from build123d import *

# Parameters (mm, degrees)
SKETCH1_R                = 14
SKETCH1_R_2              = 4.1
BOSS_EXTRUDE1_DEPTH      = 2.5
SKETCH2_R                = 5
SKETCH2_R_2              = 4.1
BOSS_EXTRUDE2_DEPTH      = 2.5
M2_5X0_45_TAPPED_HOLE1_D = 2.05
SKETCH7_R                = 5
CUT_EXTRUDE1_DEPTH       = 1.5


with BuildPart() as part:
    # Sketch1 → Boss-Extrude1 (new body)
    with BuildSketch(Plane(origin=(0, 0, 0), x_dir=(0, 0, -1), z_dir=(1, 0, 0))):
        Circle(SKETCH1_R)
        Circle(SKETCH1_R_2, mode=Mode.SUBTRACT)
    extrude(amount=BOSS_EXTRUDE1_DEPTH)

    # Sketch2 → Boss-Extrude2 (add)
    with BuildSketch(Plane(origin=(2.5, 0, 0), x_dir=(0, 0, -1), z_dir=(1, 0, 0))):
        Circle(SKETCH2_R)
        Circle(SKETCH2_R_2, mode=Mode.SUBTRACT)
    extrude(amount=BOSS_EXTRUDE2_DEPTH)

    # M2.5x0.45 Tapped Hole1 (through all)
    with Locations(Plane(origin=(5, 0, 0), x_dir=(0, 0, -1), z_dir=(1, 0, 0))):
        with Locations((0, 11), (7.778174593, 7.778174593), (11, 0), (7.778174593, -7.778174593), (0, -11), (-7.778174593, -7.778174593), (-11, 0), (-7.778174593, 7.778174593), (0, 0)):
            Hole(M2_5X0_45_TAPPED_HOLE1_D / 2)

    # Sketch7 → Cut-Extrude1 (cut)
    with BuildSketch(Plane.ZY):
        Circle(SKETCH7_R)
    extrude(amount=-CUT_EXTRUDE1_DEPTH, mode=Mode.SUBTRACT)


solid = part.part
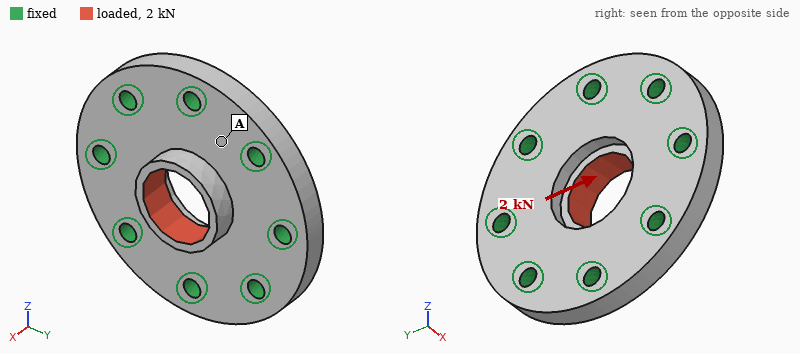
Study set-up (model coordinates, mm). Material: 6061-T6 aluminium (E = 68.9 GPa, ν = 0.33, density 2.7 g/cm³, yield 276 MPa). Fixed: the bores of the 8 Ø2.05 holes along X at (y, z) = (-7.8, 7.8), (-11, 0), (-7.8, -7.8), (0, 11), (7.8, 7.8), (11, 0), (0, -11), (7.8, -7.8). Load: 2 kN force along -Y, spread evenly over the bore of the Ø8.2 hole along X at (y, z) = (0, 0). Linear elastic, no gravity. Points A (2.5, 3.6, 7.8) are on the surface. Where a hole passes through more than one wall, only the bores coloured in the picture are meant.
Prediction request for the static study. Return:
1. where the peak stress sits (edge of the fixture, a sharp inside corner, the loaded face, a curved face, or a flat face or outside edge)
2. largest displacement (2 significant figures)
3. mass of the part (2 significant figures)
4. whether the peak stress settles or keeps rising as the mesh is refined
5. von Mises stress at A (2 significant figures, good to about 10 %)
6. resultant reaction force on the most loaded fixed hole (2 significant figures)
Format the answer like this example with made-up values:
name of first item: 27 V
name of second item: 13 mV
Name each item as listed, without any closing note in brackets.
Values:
where the peak stress sits: a sharp inside corner
largest displacement: 19 µm
mass of the part: 3.7 g
whether the peak stress settles or keeps rising as the mesh is refined: keeps rising
von Mises stress at A: 22 MPa
resultant reaction force on the most loaded fixed hole: 410 N
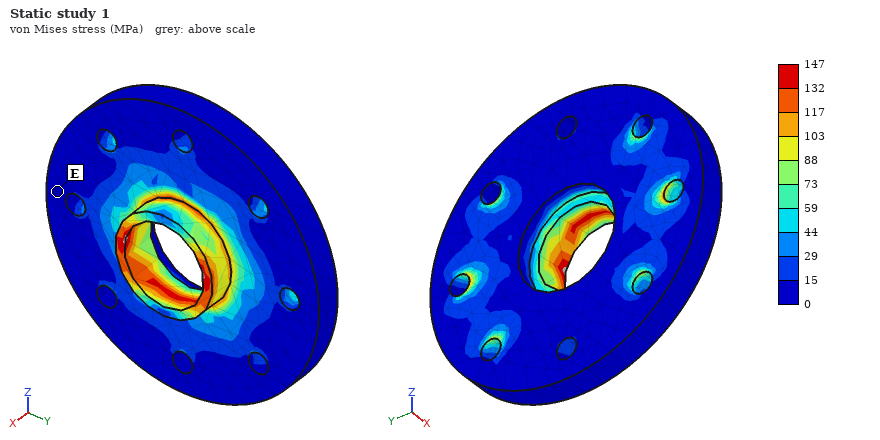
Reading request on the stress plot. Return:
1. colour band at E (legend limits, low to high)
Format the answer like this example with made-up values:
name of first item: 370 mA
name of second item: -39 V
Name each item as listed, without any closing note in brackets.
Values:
colour band at E: 0 to 15 MPa
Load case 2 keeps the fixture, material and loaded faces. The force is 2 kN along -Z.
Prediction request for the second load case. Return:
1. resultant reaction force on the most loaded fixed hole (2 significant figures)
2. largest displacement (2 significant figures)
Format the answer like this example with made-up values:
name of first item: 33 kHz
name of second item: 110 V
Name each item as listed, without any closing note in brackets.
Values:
resultant reaction force on the most loaded fixed hole: 410 N
largest displacement: 20 µm
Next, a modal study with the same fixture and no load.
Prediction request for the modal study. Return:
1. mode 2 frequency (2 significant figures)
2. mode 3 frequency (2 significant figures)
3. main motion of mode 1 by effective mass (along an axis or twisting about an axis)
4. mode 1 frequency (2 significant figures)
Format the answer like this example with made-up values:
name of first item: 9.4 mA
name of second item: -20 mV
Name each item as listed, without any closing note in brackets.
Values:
mode 2 frequency: 73 kHz
mode 3 frequency: 73 kHz
main motion of mode 1 by effective mass: along X
mode 1 frequency: 56 kHz
